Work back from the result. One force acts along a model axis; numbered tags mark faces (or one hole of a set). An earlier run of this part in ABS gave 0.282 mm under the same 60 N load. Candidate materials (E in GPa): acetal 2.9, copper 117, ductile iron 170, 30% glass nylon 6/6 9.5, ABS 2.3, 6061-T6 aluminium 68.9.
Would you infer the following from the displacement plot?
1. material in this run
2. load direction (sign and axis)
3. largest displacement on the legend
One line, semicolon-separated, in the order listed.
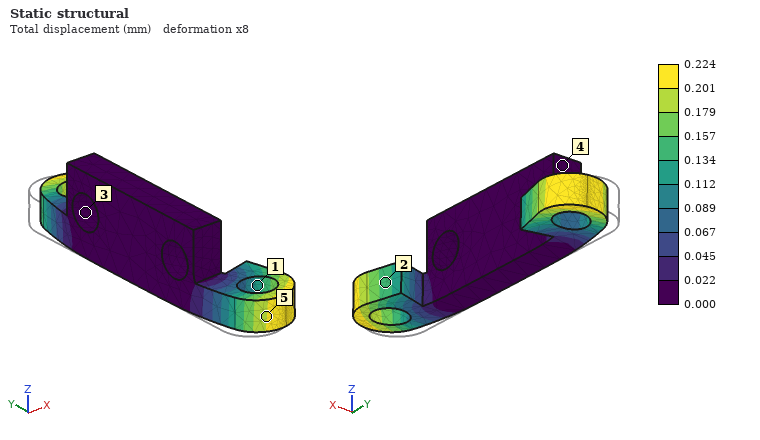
acetal; +X; 0.224 mm
